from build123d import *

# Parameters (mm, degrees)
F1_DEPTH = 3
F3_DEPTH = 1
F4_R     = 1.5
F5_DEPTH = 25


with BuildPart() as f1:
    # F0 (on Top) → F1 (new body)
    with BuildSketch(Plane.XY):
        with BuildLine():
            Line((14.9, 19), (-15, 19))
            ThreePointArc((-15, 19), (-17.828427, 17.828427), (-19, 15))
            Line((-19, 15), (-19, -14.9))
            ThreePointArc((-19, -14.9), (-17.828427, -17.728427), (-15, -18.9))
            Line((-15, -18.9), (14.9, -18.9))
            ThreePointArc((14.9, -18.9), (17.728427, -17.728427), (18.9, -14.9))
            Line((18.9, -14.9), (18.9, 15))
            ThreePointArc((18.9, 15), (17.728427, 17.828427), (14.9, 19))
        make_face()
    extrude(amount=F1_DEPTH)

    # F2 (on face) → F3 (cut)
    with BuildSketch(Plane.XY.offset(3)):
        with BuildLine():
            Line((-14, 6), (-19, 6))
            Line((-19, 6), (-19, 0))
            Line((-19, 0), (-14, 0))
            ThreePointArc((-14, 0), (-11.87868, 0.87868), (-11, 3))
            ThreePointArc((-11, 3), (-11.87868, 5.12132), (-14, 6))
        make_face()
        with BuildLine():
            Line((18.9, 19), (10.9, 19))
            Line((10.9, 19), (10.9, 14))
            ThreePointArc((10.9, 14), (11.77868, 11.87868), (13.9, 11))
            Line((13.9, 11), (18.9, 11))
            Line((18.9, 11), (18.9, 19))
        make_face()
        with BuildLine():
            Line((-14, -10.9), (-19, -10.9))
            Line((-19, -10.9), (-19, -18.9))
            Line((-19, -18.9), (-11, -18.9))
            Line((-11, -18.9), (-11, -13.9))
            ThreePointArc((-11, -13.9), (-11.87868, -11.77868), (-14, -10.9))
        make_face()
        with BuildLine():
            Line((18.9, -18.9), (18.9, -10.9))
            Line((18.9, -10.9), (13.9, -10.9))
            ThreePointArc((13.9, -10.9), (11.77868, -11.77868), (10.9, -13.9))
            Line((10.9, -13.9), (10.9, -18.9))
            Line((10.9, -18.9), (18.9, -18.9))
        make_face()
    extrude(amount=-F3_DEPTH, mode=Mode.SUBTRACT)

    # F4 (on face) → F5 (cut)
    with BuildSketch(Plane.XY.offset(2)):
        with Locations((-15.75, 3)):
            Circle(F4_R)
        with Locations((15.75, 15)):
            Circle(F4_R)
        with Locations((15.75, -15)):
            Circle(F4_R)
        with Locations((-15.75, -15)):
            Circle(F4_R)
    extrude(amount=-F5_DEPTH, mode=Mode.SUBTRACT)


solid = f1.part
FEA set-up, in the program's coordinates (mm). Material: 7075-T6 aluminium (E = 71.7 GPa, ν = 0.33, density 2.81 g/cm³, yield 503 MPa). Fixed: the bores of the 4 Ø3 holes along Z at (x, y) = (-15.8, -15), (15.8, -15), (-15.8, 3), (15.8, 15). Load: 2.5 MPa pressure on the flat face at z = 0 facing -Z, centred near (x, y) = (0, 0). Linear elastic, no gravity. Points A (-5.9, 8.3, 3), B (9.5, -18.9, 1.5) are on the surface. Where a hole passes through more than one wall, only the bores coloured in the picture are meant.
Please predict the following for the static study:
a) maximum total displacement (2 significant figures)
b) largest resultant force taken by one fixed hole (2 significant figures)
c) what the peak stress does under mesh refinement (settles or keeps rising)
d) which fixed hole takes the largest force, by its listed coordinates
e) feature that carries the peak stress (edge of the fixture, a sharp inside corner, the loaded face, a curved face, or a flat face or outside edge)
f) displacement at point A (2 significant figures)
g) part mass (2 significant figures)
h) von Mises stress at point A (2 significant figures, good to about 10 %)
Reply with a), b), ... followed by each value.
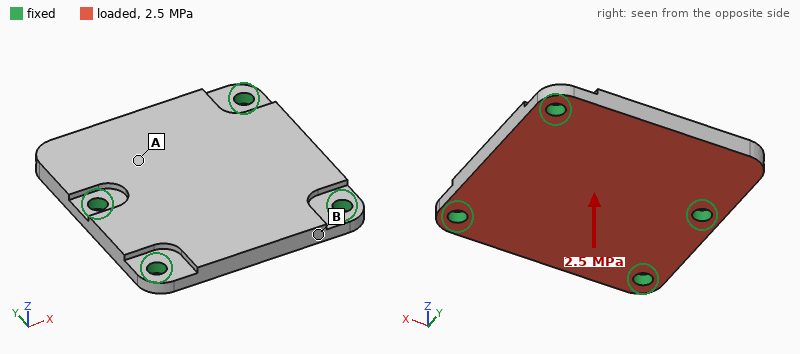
a) 0.18 mm
b) 1.4 kN
c) keeps rising
d) (-15.8, 3)
e) edge of the fixture
f) 0.100 mm
g) 11 g
h) 130 MPa
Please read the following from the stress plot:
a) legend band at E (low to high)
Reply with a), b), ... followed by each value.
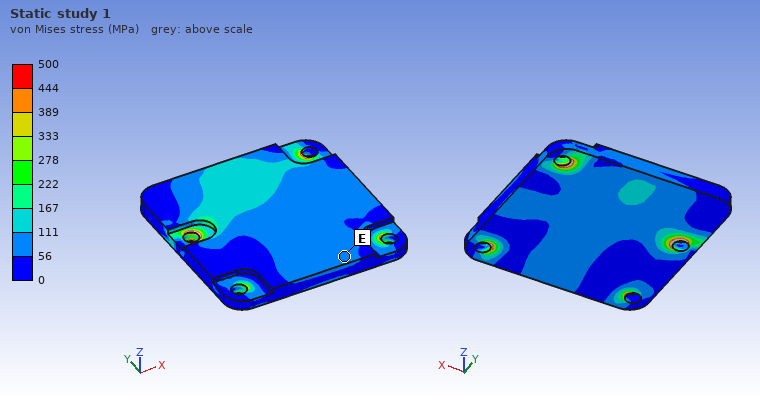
a) 56 to 111 MPa
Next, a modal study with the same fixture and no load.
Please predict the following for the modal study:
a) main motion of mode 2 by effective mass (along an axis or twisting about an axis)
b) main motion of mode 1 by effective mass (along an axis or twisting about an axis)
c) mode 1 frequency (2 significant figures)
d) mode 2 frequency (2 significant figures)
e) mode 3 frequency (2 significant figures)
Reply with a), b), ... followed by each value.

a) along Z
b) along Z
c) 8200 Hz
d) 11 kHz
e) 15 kHz
